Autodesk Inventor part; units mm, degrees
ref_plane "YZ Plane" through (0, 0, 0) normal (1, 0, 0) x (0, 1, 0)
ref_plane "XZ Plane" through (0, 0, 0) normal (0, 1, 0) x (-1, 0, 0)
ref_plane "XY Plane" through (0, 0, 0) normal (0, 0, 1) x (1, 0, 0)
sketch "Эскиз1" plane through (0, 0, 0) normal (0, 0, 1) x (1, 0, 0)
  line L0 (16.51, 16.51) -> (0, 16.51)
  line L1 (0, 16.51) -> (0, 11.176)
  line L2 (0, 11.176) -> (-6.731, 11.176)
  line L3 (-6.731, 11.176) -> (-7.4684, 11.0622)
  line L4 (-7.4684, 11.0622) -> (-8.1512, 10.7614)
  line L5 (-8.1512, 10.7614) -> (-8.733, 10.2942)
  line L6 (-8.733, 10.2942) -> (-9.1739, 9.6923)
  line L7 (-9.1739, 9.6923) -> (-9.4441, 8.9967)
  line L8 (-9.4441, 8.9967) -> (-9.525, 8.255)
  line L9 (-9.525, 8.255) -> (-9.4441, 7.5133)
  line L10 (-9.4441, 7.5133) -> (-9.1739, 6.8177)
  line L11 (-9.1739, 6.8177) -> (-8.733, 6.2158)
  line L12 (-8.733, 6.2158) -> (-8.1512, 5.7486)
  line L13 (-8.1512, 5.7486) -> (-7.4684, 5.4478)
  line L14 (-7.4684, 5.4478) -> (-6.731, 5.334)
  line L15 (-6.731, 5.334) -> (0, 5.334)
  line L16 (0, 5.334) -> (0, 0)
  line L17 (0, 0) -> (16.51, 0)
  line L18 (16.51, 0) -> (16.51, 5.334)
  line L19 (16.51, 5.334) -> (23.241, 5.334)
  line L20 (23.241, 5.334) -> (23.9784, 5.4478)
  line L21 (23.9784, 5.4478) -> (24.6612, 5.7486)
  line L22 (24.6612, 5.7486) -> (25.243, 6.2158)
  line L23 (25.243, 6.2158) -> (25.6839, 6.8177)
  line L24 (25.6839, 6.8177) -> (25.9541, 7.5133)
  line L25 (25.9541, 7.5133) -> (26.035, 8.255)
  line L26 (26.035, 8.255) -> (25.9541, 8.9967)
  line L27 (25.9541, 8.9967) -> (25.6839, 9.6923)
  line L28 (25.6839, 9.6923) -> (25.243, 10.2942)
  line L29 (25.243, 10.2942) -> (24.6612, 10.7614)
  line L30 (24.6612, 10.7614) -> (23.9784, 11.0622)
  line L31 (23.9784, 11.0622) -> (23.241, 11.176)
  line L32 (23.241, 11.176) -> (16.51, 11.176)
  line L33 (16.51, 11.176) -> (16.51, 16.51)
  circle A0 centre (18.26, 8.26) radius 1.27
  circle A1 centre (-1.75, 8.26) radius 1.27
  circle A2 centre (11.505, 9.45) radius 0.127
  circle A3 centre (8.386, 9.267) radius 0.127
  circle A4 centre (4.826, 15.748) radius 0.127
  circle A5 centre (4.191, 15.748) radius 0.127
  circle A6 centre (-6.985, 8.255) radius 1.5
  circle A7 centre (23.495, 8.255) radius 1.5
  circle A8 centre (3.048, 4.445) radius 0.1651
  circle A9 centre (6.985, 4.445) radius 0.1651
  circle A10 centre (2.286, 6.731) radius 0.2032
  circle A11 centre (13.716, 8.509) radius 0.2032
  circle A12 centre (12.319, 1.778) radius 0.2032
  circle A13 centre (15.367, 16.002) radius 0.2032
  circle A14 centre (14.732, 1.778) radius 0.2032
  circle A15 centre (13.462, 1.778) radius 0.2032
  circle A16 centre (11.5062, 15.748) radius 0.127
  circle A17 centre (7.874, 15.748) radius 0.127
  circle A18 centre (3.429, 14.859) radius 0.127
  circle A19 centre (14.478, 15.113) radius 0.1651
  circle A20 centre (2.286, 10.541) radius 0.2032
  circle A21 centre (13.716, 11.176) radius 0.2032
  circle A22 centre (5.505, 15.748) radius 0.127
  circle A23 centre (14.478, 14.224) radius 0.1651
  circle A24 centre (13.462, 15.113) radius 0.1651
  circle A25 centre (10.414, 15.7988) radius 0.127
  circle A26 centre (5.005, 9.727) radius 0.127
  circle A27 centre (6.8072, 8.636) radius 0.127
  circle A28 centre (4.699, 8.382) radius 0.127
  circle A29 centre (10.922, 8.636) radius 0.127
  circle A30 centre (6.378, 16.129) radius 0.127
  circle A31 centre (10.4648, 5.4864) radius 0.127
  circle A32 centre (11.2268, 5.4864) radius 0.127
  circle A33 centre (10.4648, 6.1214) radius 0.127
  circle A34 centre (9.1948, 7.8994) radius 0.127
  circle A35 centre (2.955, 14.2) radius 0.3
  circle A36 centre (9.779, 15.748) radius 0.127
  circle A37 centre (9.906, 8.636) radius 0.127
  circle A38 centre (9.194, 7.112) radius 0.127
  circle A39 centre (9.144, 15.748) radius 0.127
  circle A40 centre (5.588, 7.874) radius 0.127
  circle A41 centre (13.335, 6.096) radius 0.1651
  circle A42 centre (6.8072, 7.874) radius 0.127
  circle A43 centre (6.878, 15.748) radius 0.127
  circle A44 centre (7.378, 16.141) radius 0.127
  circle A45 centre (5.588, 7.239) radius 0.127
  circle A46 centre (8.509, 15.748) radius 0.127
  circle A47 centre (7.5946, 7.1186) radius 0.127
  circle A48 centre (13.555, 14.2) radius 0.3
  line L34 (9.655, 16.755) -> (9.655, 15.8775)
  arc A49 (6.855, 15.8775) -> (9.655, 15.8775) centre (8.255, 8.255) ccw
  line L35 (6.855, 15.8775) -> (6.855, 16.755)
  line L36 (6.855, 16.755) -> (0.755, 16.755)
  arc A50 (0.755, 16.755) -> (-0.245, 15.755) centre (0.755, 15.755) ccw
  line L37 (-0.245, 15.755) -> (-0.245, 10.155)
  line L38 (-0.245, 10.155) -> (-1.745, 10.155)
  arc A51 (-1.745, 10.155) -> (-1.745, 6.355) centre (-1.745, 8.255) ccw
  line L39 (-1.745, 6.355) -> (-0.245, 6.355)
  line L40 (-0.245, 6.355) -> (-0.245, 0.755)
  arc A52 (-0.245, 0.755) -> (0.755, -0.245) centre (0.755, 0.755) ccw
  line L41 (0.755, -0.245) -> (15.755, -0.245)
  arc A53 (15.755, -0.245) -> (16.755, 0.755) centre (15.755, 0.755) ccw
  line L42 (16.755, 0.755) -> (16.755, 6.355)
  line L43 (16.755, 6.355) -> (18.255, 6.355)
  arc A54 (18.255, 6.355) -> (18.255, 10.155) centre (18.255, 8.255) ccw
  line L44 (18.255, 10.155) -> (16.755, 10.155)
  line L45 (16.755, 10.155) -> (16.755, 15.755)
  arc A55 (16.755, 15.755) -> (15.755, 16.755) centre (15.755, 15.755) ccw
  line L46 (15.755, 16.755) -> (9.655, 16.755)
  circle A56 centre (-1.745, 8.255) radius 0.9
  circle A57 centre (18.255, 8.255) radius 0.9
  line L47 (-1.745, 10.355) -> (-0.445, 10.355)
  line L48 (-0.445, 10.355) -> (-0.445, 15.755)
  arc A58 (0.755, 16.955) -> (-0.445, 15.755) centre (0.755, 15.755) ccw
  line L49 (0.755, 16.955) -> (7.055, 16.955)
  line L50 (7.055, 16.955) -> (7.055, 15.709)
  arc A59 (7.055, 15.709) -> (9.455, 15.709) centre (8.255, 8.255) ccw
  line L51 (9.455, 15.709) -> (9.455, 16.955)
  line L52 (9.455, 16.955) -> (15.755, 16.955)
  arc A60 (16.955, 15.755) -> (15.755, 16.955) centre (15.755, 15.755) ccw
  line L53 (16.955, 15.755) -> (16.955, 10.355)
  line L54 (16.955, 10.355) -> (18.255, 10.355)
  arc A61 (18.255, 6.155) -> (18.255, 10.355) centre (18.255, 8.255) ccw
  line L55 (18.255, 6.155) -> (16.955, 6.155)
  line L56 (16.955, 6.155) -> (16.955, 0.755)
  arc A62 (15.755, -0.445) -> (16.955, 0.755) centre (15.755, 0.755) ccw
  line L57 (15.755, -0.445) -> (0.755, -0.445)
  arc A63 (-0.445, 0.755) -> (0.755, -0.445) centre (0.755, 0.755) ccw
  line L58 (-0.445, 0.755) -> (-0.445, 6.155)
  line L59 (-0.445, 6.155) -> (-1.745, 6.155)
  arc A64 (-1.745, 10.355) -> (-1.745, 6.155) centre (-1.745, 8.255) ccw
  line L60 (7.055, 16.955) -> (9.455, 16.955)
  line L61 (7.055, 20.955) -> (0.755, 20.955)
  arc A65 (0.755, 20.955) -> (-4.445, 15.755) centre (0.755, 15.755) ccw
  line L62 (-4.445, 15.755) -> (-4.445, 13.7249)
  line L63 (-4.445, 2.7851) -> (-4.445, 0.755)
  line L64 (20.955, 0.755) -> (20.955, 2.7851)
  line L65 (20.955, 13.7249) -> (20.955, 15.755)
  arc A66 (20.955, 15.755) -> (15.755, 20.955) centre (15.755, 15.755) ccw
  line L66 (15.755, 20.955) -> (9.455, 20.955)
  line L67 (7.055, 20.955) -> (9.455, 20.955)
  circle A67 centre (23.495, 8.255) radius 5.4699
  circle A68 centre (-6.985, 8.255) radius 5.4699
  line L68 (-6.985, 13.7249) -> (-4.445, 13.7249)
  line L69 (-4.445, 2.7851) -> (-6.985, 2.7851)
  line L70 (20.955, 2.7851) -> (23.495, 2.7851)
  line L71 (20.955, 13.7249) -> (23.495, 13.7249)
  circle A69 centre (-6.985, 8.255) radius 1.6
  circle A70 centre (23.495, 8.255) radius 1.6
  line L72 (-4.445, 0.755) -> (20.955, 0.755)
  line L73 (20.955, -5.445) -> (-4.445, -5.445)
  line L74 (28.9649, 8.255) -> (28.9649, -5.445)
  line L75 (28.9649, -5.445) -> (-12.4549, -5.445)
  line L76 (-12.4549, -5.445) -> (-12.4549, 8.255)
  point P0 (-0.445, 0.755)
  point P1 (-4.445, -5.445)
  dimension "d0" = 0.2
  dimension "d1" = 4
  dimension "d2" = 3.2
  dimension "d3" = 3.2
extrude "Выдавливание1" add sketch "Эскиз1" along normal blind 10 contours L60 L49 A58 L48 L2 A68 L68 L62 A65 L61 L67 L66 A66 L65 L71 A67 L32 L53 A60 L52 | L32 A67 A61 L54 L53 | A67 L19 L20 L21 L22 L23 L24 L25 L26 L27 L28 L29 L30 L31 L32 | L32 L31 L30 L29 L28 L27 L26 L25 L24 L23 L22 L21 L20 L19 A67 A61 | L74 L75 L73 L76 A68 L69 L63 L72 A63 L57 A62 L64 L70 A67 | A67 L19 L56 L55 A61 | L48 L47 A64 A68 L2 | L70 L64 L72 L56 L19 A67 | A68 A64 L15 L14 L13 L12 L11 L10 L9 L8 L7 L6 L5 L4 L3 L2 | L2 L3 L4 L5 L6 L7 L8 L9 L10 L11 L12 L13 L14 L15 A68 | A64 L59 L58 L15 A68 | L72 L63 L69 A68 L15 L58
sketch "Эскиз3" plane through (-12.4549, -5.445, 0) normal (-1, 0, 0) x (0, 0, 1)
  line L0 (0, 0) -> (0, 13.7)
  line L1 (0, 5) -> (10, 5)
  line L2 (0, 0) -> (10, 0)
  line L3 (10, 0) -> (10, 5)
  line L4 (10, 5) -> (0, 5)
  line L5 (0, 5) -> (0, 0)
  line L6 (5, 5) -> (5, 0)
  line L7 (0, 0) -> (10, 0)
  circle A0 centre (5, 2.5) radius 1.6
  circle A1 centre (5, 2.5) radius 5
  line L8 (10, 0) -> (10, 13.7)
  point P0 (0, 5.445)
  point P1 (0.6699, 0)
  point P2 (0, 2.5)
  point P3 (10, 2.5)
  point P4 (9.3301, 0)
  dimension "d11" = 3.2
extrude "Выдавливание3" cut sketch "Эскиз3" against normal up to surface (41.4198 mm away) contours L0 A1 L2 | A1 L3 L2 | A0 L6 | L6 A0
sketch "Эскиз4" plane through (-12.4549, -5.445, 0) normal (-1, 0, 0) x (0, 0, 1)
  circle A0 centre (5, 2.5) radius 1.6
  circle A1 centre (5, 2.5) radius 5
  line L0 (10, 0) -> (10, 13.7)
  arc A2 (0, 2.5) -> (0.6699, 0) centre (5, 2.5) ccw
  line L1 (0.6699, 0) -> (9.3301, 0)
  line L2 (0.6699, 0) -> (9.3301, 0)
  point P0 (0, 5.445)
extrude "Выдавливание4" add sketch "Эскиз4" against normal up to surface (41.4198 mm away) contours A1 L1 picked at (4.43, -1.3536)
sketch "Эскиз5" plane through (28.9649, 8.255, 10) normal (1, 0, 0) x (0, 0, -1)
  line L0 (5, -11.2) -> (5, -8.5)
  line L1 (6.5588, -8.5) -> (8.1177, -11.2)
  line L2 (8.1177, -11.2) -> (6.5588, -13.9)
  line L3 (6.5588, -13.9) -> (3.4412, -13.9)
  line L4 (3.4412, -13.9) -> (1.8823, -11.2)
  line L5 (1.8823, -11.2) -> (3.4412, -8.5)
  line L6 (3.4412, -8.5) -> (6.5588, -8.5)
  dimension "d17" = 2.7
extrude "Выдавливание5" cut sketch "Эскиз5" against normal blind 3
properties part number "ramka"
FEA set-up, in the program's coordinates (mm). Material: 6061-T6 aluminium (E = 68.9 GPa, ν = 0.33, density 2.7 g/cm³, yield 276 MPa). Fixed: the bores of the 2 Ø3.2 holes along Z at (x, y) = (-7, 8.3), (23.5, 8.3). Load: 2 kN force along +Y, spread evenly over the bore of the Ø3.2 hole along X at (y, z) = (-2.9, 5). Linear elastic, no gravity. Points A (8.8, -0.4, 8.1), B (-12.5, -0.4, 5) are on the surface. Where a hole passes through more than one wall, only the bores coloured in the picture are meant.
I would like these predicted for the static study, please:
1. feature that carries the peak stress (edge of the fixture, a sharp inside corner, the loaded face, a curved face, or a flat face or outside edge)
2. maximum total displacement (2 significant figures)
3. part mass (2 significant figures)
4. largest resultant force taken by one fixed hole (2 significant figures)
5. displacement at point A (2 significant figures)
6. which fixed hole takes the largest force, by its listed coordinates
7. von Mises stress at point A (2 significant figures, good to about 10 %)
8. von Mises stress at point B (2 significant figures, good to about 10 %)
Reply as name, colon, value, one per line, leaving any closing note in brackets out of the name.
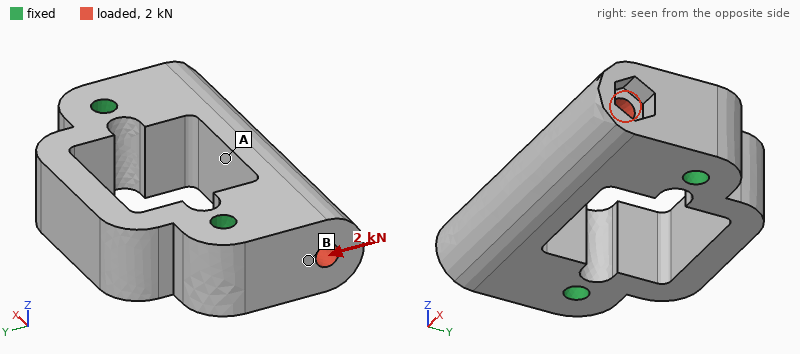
feature that carries the peak stress: a curved face
maximum total displacement: 7.8 µm
part mass: 17 g
largest resultant force taken by one fixed hole: 1.1 kN
displacement at point A: 7.1 µm
which fixed hole takes the largest force, by its listed coordinates: (-7, 8.3)
von Mises stress at point A: 12 MPa
von Mises stress at point B: 5.0 MPa
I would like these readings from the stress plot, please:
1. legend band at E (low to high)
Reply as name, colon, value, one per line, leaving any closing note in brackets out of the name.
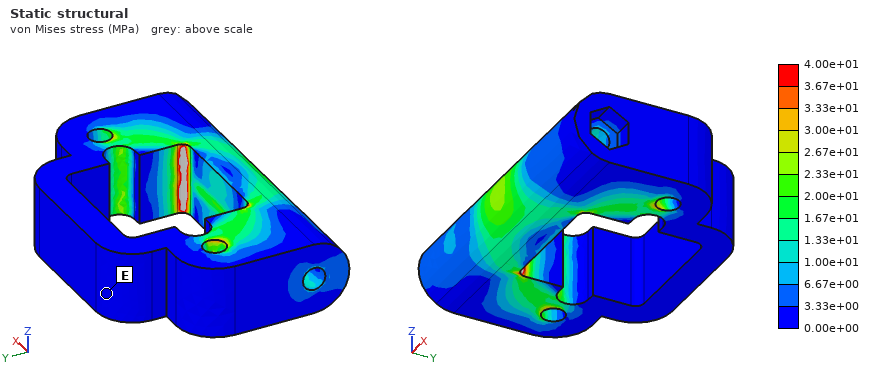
legend band at E: 0.00e+00 to 3.33e+00 MPa
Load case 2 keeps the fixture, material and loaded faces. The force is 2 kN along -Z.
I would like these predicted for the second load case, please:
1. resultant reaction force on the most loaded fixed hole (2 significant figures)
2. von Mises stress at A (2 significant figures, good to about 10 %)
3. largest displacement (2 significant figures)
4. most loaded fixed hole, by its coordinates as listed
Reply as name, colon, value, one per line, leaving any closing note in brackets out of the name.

resultant reaction force on the most loaded fixed hole: 1.1 kN
von Mises stress at A: 13 MPa
largest displacement: 27 µm
most loaded fixed hole, by its coordinates as listed: (-7, 8.3)
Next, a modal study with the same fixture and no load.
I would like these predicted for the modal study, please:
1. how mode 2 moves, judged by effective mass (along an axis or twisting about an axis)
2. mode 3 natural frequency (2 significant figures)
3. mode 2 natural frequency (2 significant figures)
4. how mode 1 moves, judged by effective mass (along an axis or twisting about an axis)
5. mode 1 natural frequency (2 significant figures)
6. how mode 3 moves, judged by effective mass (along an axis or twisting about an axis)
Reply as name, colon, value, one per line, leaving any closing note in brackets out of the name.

how mode 2 moves, judged by effective mass: along X
mode 3 natural frequency: 22 kHz
mode 2 natural frequency: 22 kHz
how mode 1 moves, judged by effective mass: along Z
mode 1 natural frequency: 19 kHz
how mode 3 moves, judged by effective mass: along Z
